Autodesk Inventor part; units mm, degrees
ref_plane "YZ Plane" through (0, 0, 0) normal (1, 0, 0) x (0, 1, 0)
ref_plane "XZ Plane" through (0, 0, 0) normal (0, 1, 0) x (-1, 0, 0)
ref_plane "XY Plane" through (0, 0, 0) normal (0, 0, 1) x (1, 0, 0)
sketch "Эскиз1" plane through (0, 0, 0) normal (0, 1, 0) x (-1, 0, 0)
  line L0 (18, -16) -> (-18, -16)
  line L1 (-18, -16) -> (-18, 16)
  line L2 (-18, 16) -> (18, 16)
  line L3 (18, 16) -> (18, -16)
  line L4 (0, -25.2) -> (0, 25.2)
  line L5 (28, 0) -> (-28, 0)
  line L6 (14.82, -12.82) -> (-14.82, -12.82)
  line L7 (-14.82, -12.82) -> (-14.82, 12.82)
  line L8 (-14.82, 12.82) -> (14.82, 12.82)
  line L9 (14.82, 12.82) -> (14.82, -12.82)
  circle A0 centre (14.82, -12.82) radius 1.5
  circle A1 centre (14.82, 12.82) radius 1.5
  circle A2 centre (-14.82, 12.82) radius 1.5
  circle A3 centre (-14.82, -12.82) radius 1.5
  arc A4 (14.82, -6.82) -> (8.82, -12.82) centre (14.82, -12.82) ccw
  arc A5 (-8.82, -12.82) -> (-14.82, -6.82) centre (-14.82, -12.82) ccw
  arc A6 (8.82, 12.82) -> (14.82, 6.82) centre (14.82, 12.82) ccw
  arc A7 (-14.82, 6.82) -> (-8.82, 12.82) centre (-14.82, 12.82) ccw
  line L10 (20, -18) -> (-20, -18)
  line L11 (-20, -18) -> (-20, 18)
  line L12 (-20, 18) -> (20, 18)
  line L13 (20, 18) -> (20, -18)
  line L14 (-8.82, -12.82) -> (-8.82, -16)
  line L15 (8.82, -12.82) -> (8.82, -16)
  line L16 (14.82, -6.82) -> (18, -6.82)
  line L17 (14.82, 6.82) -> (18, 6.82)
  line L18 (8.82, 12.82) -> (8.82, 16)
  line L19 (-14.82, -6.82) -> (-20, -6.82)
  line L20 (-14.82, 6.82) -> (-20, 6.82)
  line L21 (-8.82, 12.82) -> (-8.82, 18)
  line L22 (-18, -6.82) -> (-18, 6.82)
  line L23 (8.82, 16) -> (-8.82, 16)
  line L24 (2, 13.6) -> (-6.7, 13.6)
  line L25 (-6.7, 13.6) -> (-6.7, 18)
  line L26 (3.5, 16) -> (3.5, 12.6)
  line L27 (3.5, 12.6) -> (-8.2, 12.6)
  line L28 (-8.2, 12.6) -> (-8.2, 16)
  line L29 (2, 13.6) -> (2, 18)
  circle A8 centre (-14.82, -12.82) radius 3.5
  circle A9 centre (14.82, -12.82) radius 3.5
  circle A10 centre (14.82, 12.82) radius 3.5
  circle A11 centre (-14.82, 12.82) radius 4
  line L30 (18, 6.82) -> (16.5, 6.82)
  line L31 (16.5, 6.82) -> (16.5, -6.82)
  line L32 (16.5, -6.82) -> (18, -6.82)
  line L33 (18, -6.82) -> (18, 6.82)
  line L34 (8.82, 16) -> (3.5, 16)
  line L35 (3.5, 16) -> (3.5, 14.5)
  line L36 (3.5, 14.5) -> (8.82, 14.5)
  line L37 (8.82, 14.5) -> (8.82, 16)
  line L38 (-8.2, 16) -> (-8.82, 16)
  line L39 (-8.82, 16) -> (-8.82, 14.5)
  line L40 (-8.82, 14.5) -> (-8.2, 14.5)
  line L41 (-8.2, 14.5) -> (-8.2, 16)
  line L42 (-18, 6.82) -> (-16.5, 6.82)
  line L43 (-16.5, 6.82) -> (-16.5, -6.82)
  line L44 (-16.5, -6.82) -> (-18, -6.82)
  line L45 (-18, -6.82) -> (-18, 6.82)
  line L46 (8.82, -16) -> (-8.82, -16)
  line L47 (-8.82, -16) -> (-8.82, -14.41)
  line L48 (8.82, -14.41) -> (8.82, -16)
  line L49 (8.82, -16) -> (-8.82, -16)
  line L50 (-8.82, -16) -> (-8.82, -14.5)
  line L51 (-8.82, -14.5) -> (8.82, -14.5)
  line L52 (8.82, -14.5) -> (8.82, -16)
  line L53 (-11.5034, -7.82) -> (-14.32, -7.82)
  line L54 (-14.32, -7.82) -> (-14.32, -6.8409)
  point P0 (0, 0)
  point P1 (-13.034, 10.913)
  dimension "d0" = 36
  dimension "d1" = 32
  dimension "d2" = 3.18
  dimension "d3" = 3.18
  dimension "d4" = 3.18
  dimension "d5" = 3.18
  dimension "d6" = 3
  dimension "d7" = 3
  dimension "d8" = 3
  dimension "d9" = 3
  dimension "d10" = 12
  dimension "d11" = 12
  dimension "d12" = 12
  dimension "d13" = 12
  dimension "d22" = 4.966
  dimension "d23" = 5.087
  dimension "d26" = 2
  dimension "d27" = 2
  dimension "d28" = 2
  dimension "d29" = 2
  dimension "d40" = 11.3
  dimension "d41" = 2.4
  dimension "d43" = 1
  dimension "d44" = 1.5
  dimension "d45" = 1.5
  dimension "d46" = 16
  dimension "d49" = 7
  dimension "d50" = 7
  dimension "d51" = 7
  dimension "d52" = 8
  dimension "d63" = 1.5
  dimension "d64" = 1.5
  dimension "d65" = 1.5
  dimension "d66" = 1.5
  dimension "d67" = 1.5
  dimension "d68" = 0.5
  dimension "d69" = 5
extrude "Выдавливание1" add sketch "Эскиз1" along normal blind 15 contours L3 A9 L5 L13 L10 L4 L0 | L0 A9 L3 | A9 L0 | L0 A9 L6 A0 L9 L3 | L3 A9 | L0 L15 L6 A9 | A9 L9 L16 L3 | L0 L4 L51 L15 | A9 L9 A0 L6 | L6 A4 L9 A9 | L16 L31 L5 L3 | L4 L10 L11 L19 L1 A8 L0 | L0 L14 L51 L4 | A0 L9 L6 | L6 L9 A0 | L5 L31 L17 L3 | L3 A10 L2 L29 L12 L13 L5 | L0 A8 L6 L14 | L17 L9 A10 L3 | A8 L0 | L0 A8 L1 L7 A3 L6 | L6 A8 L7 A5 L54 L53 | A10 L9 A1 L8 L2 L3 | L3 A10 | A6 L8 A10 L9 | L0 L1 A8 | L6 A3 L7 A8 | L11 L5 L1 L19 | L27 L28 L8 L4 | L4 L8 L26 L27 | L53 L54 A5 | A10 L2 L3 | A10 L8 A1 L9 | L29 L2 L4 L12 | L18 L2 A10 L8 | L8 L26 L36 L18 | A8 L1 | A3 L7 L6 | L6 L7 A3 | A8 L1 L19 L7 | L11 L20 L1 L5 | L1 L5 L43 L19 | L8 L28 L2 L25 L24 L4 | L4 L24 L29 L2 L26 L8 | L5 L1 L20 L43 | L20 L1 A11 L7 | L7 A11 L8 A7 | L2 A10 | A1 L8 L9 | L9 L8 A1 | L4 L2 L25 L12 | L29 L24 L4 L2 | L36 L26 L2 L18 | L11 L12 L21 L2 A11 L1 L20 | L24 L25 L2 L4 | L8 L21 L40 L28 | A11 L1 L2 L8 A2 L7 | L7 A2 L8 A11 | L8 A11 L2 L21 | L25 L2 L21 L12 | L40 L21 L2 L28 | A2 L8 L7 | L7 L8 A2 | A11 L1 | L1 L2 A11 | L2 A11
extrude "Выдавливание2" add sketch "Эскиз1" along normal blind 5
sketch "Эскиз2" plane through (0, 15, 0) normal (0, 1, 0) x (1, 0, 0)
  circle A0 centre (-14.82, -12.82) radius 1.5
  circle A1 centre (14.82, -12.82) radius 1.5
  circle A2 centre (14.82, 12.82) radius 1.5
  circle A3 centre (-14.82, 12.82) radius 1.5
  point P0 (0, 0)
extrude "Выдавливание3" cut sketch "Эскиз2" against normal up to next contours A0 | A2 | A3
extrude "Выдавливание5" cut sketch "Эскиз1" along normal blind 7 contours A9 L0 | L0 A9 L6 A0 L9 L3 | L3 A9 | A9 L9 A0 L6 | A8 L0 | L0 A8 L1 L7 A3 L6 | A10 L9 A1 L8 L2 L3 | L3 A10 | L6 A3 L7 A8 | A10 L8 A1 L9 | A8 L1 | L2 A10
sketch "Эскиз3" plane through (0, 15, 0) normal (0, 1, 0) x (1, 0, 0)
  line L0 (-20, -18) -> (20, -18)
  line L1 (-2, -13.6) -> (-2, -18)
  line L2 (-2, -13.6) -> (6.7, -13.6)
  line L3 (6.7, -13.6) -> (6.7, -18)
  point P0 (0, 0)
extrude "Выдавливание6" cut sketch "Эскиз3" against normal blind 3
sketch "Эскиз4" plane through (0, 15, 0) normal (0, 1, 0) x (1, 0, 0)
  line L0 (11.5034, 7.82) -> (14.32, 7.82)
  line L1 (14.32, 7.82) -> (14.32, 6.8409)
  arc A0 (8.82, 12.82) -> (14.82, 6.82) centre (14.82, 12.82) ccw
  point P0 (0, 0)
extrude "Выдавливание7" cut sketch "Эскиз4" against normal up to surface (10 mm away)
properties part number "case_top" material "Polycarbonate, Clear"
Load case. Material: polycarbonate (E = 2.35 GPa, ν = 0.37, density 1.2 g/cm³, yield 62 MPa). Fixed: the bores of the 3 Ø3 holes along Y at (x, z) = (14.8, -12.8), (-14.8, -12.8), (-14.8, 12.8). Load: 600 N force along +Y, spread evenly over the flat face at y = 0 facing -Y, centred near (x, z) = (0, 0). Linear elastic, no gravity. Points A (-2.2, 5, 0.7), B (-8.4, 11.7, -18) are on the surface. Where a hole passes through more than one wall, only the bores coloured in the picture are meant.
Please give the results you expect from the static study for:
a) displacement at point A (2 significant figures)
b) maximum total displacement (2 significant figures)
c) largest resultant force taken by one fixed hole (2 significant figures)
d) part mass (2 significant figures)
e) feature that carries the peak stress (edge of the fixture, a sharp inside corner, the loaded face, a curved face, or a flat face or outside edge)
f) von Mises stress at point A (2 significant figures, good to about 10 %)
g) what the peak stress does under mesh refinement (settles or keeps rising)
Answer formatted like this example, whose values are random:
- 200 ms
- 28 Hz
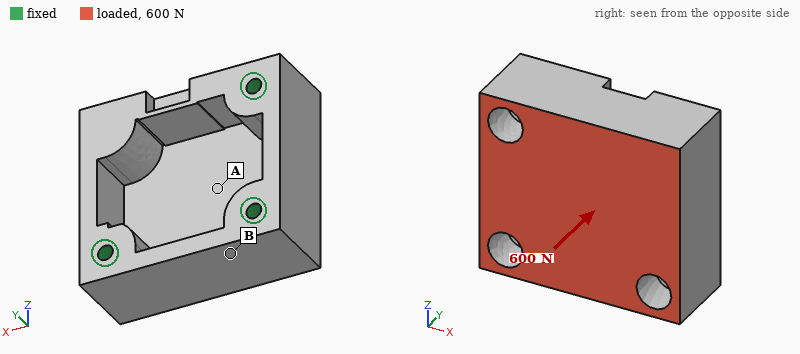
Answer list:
- 0.073 mm
- 0.19 mm
- 300 N
- 16 g
- edge of the fixture
- 2.8 MPa
- keeps rising
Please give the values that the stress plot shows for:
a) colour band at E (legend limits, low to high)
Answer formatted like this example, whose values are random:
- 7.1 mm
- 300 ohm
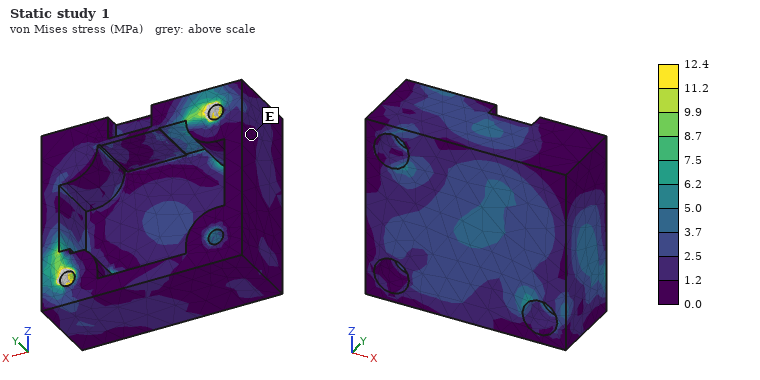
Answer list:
- 0.0 to 1.2 MPa
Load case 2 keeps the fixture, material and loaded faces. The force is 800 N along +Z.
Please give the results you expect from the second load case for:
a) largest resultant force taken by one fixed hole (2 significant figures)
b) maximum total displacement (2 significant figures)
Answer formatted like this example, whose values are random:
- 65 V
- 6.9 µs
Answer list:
- 360 N
- 0.20 mm
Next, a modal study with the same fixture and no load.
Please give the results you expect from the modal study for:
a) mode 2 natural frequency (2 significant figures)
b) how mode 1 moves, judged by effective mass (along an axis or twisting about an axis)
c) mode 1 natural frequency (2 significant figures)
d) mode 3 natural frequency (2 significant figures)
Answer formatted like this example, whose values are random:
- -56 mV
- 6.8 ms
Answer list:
- 5200 Hz
- along Y
- 2700 Hz
- 6200 Hz
